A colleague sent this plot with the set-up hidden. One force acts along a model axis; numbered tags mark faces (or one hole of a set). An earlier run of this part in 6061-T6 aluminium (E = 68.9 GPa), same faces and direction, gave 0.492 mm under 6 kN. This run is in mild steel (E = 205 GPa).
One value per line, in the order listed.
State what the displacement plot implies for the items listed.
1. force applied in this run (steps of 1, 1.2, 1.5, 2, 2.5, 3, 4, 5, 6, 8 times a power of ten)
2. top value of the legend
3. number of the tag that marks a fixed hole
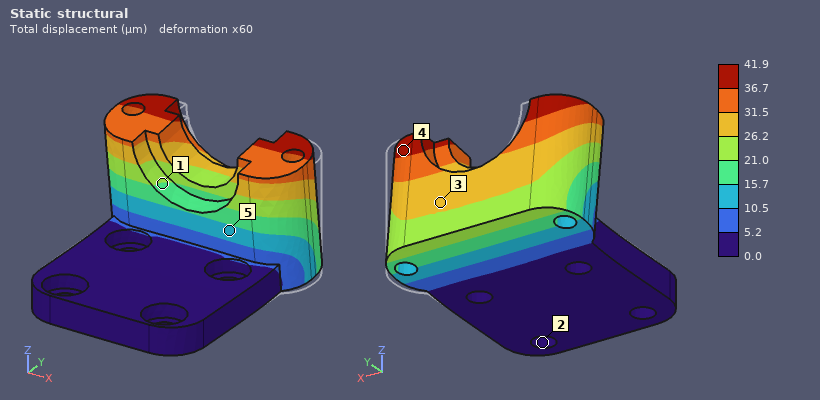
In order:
1.5 kN
41.9 µm
2
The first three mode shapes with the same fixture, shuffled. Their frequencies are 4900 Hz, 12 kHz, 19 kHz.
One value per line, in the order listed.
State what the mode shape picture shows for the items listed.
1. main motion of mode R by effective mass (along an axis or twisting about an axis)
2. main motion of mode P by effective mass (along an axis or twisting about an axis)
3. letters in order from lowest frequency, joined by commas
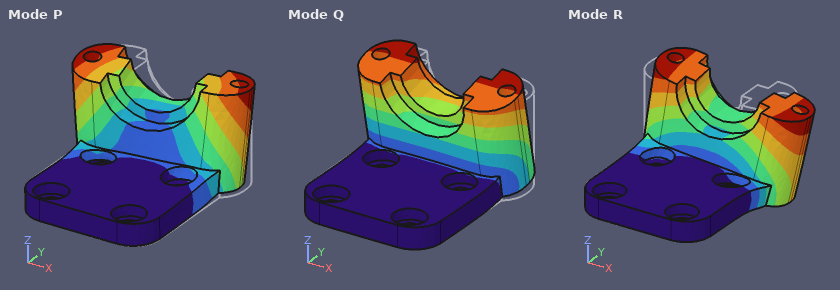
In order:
along X
along X
Q, R, P
